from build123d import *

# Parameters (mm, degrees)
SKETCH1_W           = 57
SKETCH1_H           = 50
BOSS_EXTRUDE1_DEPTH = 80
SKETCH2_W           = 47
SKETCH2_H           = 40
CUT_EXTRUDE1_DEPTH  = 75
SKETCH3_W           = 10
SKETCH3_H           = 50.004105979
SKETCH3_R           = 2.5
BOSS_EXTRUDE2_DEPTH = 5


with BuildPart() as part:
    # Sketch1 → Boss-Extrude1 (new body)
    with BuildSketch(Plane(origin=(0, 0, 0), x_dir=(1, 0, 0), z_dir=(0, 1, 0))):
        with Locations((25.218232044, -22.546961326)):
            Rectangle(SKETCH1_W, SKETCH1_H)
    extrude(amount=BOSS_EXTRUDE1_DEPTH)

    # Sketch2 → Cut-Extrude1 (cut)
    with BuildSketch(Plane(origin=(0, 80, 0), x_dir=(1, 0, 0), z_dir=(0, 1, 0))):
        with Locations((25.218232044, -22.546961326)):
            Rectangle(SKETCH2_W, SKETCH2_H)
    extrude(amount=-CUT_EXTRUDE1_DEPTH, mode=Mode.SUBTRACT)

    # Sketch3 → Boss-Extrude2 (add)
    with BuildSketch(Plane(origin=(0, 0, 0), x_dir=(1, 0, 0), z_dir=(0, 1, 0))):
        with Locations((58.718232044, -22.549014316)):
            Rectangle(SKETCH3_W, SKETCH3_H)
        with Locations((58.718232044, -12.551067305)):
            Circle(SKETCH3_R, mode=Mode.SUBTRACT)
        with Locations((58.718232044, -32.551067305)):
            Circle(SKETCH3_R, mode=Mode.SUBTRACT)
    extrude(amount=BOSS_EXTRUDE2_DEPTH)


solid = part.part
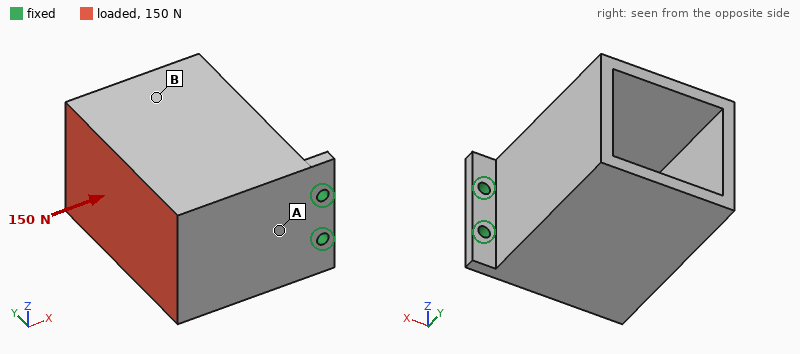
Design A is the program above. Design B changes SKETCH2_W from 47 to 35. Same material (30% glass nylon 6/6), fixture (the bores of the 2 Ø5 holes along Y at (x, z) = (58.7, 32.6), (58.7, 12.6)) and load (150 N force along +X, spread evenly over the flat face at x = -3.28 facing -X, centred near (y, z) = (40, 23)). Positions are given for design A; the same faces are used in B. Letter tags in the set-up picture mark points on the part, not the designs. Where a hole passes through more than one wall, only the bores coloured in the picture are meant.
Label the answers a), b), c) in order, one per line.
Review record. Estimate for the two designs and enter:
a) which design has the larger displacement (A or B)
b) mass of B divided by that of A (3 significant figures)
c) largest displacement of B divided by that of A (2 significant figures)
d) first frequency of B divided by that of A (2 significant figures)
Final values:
a) A
b) 1.40
c) 0.88
d) 0.87
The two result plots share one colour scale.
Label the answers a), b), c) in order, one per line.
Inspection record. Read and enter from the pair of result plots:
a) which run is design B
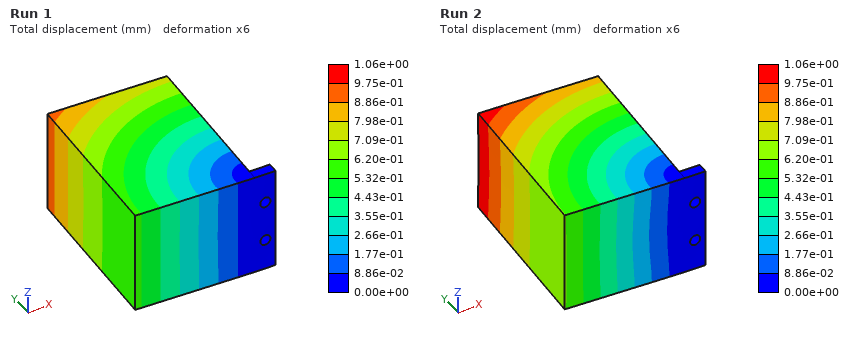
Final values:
a) Run 1
